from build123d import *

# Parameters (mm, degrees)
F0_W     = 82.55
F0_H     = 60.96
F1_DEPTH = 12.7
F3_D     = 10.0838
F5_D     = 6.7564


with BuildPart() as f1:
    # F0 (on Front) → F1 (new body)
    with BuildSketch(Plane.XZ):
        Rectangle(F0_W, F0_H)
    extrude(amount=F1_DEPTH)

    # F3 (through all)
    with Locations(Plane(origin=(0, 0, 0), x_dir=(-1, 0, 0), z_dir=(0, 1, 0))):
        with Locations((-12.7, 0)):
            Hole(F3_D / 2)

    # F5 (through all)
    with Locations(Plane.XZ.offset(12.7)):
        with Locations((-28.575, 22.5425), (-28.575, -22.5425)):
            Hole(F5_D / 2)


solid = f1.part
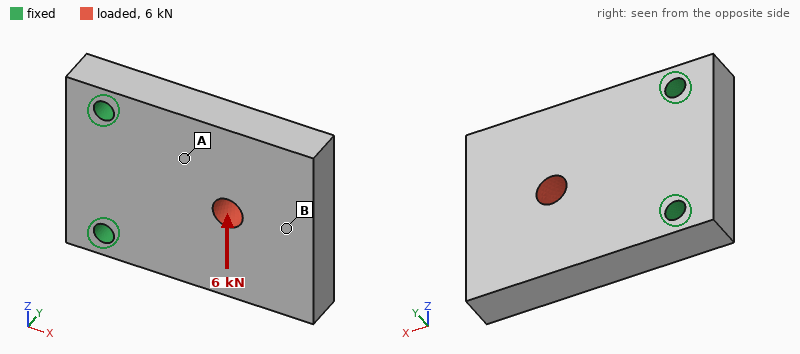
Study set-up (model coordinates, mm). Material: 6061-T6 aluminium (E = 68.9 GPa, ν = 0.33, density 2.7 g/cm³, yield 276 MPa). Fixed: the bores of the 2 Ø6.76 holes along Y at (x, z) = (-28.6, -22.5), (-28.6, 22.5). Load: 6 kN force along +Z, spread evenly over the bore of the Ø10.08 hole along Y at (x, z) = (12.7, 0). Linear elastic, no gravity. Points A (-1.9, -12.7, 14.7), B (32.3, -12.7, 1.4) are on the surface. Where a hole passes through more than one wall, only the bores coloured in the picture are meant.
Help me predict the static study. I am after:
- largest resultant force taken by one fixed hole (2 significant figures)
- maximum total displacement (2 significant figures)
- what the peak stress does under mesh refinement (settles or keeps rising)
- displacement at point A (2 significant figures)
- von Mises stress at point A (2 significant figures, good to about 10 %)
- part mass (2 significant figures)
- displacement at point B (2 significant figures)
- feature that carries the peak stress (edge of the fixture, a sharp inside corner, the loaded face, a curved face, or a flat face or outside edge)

5.9 kN
35 µm
keeps rising
14 µm
17 MPa
170 g
30 µm
edge of the fixture
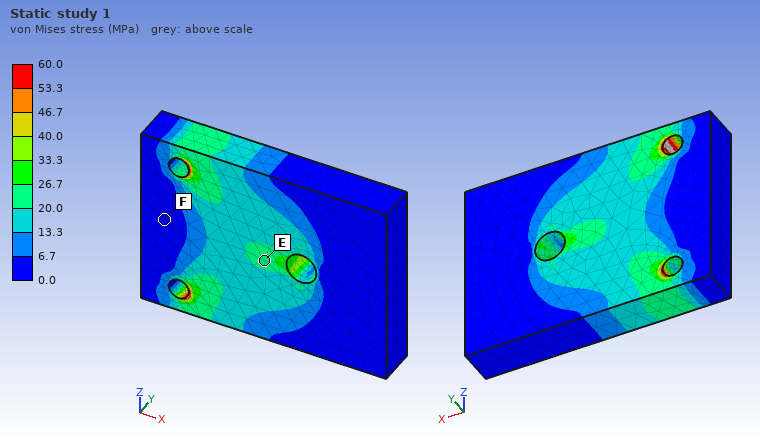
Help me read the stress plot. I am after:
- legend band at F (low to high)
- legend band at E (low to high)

0.0 to 6.7 MPa
20.0 to 26.7 MPa
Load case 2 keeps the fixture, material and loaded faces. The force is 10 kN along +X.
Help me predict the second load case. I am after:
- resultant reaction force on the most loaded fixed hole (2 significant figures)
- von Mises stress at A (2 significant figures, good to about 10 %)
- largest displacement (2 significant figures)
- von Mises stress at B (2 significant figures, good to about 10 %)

5.1 kN
15 MPa
15 µm
7.7 MPa
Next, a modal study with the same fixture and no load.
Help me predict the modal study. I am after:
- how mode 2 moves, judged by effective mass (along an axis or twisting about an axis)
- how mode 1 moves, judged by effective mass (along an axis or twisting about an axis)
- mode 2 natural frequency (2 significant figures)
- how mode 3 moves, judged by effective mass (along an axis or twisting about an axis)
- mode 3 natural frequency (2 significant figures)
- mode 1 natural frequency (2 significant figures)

twisting about X
along Y
5100 Hz
along Z
6900 Hz
2000 Hz
